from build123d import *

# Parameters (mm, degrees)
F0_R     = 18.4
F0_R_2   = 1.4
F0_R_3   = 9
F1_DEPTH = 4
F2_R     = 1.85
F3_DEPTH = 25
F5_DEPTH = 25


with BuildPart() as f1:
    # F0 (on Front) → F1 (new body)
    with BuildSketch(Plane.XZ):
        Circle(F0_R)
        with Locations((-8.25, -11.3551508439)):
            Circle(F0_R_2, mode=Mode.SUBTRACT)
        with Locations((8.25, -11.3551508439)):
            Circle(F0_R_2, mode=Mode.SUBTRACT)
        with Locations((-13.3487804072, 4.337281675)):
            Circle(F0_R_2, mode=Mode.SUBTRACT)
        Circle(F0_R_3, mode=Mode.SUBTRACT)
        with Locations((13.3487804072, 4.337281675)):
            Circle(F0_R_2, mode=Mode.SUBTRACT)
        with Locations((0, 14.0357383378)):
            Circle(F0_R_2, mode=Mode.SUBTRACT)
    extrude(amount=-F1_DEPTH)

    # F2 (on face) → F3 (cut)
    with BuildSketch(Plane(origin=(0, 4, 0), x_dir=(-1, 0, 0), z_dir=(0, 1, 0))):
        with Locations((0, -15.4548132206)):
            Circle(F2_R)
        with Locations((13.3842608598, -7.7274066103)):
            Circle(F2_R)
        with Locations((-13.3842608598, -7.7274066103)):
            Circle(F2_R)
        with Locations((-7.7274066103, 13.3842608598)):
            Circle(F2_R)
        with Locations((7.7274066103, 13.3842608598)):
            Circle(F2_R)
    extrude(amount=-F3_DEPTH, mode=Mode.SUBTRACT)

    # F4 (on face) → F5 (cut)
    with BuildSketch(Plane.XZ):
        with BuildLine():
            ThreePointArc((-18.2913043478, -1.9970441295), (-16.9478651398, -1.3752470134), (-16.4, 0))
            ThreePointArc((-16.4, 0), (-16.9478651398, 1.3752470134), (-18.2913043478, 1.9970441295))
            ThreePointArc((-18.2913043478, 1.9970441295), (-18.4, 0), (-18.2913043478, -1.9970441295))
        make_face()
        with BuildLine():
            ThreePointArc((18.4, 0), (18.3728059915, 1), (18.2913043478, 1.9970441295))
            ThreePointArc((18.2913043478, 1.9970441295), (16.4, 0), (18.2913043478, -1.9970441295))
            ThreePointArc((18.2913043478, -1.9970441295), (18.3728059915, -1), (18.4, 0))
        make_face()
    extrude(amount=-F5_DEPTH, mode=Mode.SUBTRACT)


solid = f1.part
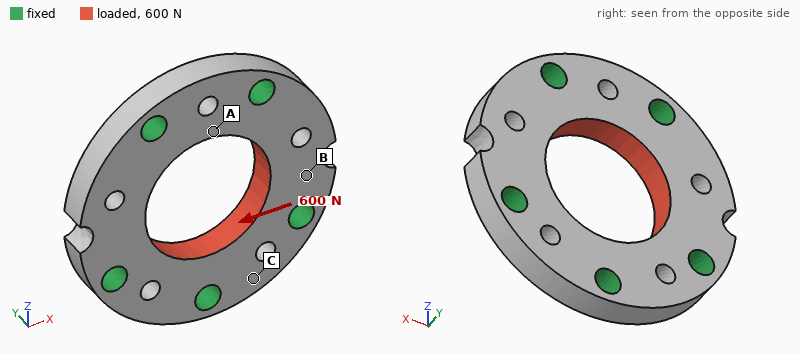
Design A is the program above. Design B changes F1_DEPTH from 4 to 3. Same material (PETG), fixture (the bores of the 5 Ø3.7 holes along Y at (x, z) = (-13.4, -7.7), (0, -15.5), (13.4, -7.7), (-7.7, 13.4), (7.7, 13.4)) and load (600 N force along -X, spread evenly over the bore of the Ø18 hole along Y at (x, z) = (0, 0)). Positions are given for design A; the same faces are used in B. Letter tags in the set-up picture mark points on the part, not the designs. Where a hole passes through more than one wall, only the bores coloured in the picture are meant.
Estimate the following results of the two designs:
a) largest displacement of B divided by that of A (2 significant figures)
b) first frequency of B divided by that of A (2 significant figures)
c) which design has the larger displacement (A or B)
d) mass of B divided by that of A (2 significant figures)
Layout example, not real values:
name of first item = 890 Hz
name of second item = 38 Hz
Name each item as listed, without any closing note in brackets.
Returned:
largest displacement of B divided by that of A = 1.3
first frequency of B divided by that of A = 0.82
which design has the larger displacement = B
mass of B divided by that of A = 0.75
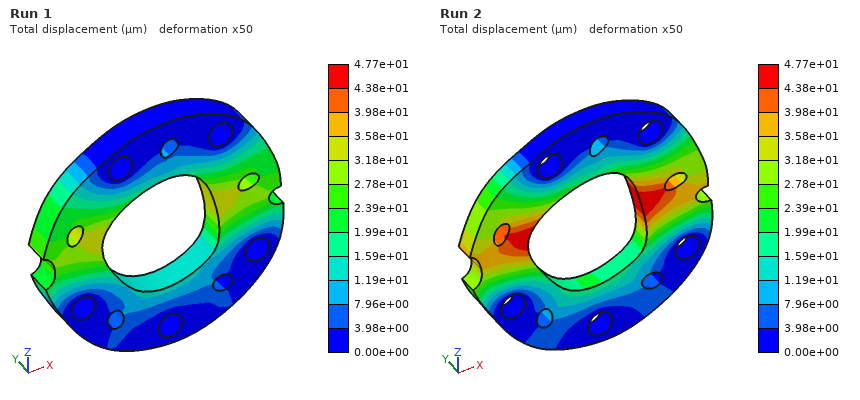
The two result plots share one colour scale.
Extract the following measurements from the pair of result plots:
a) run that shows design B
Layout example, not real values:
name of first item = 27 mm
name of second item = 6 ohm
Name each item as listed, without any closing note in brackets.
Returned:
run that shows design B = Run 2
